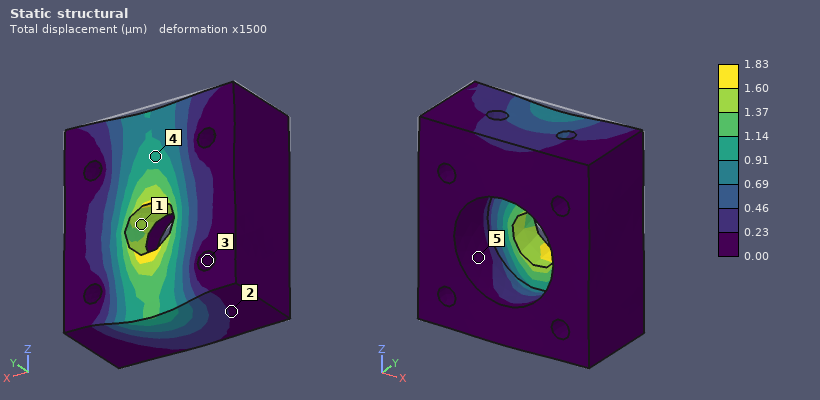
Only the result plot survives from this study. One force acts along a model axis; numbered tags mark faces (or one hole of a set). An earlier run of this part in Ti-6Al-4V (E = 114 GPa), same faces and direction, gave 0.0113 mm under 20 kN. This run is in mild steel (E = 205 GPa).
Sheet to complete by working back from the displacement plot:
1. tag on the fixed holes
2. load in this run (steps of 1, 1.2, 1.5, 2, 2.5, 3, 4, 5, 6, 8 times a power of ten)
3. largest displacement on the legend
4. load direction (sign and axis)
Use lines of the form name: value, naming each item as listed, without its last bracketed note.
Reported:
tag on the fixed holes: 3
load in this run: 6 kN
largest displacement on the legend: 1.83 µm
load direction: -Z
